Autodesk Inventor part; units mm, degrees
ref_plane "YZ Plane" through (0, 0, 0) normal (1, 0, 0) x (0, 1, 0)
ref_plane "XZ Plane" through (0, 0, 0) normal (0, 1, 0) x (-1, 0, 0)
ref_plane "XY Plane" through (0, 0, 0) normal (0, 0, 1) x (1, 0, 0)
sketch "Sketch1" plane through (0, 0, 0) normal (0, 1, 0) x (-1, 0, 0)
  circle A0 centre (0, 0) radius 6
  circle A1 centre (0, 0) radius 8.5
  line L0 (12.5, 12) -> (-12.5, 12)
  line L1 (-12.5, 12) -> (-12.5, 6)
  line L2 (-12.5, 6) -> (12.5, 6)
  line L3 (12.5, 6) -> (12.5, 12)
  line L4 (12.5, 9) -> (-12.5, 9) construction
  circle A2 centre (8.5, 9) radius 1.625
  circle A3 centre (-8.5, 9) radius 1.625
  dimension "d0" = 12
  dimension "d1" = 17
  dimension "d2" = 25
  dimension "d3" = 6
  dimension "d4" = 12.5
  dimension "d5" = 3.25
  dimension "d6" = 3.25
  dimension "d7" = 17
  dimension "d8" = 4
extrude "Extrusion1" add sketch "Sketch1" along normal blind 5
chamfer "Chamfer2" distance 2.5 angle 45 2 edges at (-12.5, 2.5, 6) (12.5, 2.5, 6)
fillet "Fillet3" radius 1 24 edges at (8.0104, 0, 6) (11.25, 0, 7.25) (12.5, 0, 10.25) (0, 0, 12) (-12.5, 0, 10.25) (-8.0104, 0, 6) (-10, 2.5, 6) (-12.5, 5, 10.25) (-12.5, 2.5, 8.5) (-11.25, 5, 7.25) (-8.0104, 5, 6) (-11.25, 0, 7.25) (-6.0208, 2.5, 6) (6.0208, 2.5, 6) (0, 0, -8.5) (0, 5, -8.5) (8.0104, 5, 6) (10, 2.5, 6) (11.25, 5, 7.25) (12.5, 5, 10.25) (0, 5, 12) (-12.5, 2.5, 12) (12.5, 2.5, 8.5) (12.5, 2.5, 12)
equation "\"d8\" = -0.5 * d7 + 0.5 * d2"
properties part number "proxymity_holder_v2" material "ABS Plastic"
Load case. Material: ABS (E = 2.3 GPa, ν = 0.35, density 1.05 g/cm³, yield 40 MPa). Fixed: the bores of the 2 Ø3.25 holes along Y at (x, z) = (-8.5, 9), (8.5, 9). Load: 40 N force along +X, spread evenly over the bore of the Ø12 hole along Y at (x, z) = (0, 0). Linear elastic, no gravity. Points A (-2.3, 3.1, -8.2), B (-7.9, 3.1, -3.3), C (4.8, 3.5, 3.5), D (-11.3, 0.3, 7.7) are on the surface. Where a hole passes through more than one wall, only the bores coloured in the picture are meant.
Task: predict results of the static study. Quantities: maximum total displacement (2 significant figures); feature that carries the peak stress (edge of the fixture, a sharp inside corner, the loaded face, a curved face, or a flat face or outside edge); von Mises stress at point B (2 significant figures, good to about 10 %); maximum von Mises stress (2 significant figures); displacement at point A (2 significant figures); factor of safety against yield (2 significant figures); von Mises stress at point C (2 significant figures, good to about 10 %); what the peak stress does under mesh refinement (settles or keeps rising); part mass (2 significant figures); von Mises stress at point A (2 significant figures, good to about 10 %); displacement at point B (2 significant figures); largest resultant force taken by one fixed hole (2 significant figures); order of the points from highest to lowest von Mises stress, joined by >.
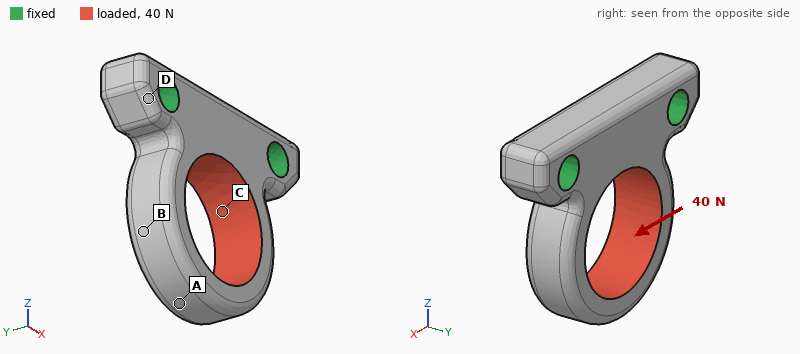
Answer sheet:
0.12 mm
a curved face
3.8 MPa
16 MPa
0.12 mm
2.5
8.8 MPa
settles
1.1 g
2.2 MPa
0.10 mm
29 N
C > B > A > D
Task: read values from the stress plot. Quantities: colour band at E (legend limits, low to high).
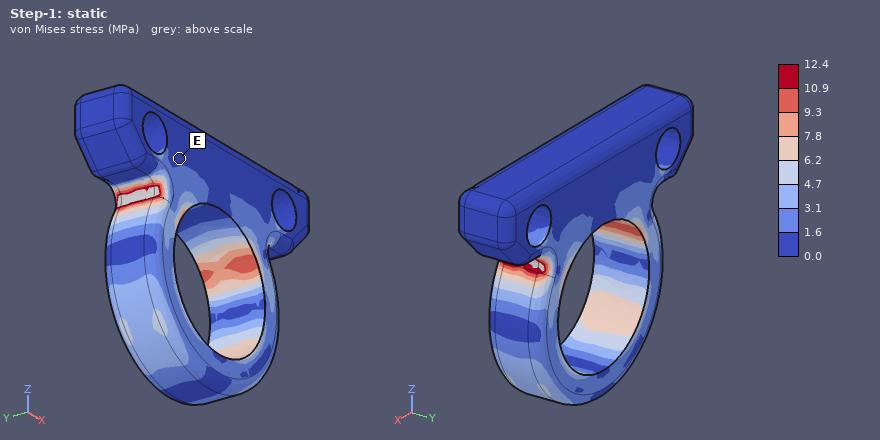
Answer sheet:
0.0 to 1.6 MPa
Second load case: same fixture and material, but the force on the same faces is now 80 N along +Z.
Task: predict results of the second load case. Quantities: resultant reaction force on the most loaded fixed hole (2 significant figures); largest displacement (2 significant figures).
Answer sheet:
41 N
38 µm
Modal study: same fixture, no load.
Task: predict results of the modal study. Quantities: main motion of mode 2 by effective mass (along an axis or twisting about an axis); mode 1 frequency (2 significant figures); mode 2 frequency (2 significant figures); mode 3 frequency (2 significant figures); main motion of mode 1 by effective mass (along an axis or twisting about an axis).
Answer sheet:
along X
3300 Hz
4200 Hz
7600 Hz
along Y
